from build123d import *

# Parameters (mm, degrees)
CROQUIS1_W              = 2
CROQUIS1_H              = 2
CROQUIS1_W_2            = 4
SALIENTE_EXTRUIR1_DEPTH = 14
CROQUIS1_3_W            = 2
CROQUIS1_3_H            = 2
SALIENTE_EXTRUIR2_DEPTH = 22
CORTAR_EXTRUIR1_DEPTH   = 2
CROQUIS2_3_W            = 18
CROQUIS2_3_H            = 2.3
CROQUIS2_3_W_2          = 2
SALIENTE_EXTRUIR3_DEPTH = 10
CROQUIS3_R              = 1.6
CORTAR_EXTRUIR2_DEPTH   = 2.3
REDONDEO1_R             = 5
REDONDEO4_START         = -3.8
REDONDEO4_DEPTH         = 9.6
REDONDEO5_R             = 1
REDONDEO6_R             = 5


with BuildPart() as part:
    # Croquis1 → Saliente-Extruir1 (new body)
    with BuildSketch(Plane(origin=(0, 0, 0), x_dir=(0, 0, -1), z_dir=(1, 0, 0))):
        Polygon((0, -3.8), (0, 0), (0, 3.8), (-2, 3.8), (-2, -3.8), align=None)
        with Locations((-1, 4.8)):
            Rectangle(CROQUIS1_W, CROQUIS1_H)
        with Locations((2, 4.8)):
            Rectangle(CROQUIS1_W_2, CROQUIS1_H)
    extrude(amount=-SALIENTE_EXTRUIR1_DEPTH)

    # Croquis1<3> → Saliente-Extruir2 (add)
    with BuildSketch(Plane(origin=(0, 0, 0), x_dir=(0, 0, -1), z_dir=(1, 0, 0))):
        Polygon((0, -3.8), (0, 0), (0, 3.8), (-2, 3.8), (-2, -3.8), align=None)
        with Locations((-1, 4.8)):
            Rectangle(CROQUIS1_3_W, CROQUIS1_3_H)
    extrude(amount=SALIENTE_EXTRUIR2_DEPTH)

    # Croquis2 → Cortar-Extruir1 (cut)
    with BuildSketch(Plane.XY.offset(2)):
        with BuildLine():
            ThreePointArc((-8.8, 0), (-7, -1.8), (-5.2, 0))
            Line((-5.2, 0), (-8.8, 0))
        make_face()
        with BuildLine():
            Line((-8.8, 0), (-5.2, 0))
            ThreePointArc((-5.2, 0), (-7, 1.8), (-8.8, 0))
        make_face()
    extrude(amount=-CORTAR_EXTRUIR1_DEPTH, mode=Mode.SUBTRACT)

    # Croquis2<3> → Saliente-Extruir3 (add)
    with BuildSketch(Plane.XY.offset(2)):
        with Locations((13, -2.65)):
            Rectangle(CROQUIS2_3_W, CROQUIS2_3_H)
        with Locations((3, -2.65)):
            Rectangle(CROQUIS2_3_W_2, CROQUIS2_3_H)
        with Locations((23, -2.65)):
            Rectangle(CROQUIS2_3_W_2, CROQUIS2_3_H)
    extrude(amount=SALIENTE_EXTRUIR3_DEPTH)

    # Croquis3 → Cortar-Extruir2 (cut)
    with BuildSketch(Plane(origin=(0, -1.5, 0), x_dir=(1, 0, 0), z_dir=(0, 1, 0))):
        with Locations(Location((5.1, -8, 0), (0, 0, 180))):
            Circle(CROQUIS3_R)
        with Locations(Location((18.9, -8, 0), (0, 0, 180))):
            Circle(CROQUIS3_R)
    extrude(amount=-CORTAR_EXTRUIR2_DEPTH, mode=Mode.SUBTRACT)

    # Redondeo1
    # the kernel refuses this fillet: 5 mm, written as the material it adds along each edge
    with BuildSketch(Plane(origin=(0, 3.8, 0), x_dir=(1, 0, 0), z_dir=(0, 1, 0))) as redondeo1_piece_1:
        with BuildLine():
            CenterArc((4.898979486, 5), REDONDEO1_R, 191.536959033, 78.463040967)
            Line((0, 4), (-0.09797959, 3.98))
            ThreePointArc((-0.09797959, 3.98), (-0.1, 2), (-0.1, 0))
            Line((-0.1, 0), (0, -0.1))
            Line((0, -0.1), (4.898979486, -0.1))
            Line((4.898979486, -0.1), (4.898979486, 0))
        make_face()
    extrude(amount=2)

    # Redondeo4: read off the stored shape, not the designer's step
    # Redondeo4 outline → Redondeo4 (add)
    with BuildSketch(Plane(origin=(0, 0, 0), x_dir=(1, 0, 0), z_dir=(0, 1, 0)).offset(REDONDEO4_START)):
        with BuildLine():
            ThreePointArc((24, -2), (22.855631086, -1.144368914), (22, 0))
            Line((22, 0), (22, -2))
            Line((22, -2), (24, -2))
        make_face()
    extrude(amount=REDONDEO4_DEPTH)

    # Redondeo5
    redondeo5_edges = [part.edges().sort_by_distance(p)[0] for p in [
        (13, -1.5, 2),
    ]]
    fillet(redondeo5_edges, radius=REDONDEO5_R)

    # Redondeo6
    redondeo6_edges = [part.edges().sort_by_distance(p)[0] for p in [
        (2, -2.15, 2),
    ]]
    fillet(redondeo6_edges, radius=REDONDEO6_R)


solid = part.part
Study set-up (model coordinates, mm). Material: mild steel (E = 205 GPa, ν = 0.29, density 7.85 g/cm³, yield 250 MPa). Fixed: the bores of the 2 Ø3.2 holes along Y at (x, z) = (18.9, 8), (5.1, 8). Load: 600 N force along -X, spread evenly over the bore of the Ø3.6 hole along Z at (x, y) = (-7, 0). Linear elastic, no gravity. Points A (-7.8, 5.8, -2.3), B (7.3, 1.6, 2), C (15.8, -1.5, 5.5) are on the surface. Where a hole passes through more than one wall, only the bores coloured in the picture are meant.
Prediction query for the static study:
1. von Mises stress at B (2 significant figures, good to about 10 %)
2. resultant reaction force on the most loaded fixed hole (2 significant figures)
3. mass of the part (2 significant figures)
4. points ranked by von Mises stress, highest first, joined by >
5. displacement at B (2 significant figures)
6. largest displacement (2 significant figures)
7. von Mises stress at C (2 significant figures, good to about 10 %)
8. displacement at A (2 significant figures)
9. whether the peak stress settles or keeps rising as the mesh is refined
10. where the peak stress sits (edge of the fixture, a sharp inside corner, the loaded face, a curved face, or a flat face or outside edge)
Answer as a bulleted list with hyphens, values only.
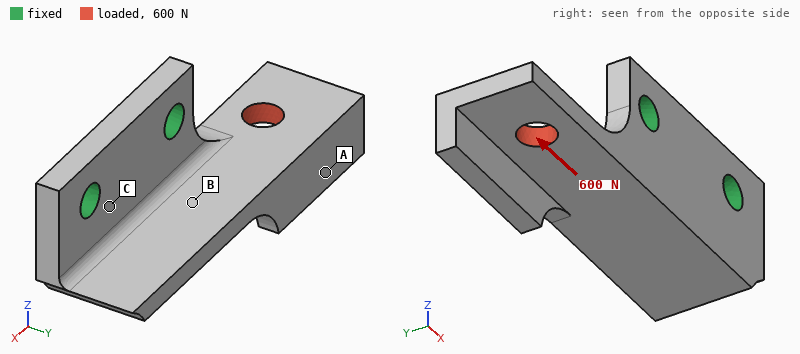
- 18 MPa
- 400 N
- 10 g
- C > B > A
- 3.7 µm
- 11 µm
- 40 MPa
- 9.3 µm
- keeps rising
- edge of the fixture
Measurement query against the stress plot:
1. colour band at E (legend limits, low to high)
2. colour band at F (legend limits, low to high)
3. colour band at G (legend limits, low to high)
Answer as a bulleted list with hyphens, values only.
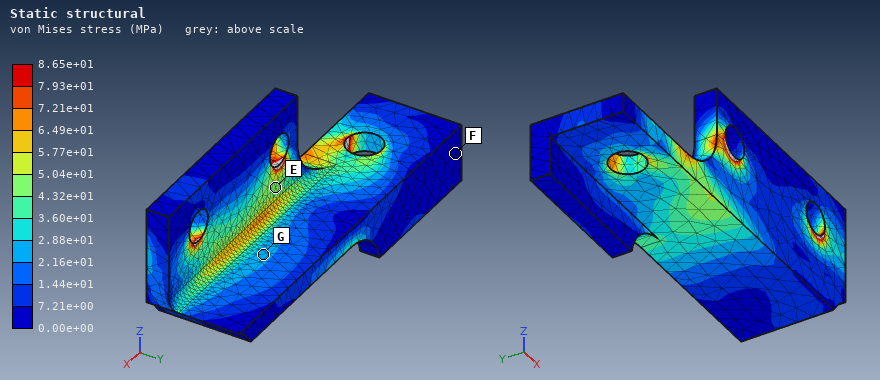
- 4.32e+01 to 5.04e+01 MPa
- 0.00e+00 to 7.21e+00 MPa
- 2.16e+01 to 2.88e+01 MPa
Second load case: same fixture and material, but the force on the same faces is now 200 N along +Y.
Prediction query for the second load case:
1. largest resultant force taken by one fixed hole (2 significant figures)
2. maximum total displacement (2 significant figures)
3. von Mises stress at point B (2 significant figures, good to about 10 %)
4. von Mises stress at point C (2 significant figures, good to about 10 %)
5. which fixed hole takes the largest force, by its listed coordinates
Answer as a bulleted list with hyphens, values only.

- 340 N
- 60 µm
- 44 MPa
- 30 MPa
- (5.1, 8)
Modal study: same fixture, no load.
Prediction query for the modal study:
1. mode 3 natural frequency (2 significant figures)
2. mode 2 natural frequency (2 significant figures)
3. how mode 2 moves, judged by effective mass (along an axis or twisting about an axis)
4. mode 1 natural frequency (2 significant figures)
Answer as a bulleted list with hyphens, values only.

- 12 kHz
- 7700 Hz
- along Y
- 4400 Hz
